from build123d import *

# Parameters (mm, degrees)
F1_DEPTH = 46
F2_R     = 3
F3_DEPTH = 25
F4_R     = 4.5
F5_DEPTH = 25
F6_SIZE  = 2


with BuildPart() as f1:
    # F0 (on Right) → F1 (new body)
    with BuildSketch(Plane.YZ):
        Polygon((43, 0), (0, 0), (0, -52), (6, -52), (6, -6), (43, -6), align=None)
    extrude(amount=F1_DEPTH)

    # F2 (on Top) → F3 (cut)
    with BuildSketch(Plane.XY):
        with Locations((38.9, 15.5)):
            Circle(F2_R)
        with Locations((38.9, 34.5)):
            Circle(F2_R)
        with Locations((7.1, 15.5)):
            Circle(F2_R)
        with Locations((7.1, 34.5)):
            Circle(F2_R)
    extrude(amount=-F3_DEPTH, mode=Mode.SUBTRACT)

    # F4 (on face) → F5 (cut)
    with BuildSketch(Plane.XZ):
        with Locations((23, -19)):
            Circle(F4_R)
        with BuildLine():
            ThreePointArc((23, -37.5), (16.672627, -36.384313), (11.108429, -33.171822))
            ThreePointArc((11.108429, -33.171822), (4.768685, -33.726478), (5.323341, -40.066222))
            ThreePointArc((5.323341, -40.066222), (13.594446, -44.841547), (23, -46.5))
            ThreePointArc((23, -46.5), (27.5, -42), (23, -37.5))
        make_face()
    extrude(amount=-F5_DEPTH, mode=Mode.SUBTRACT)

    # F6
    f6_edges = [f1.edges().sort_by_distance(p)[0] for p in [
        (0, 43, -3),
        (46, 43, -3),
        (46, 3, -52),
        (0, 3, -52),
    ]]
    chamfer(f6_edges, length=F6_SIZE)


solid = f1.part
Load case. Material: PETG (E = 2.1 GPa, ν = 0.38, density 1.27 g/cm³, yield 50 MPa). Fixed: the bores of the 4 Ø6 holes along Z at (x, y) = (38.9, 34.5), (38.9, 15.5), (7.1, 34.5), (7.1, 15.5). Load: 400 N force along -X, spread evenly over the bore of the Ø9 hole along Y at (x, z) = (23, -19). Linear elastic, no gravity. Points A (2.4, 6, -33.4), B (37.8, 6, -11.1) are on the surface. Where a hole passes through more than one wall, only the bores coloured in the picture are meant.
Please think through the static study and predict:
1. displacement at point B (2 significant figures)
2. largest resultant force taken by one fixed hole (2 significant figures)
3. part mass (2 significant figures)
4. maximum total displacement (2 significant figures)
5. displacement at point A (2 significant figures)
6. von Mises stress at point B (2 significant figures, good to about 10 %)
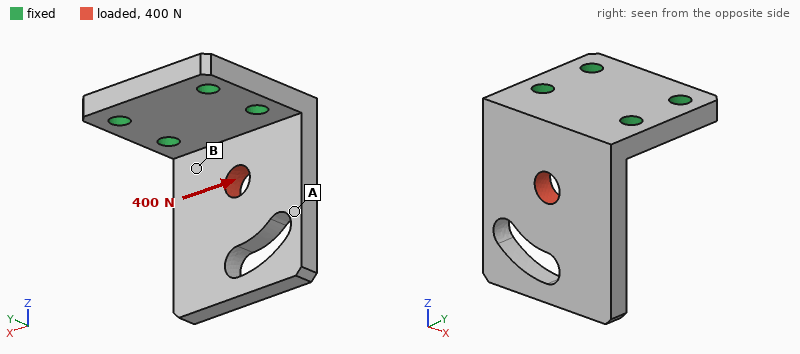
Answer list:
0.12 mm
300 N
28 g
0.41 mm
0.31 mm
5.6 MPa
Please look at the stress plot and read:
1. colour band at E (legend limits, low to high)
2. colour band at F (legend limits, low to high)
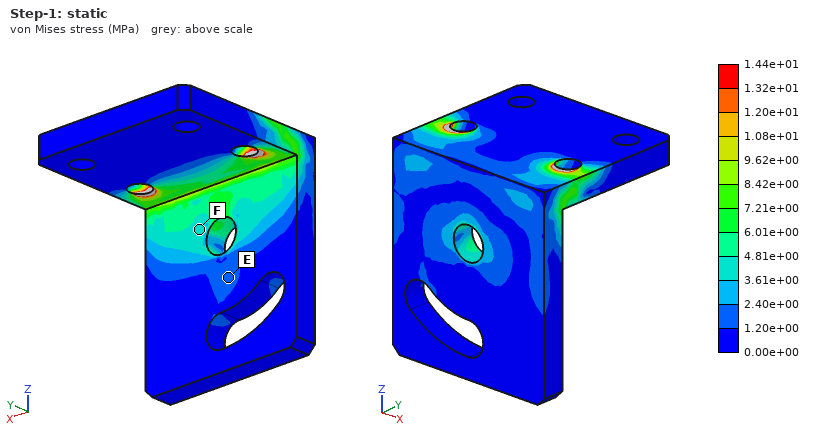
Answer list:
1.20e+00 to 2.40e+00 MPa
3.61e+00 to 4.81e+00 MPa
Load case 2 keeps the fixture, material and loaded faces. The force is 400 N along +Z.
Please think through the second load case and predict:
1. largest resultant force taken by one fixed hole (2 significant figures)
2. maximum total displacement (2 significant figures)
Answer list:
230 N
0.82 mm
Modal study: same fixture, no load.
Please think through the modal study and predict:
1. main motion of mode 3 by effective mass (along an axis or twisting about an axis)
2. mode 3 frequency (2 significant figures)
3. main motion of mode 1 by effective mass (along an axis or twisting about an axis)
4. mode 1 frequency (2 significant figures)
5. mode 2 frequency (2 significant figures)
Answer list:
along X
1400 Hz
along Y
420 Hz
1000 Hz
